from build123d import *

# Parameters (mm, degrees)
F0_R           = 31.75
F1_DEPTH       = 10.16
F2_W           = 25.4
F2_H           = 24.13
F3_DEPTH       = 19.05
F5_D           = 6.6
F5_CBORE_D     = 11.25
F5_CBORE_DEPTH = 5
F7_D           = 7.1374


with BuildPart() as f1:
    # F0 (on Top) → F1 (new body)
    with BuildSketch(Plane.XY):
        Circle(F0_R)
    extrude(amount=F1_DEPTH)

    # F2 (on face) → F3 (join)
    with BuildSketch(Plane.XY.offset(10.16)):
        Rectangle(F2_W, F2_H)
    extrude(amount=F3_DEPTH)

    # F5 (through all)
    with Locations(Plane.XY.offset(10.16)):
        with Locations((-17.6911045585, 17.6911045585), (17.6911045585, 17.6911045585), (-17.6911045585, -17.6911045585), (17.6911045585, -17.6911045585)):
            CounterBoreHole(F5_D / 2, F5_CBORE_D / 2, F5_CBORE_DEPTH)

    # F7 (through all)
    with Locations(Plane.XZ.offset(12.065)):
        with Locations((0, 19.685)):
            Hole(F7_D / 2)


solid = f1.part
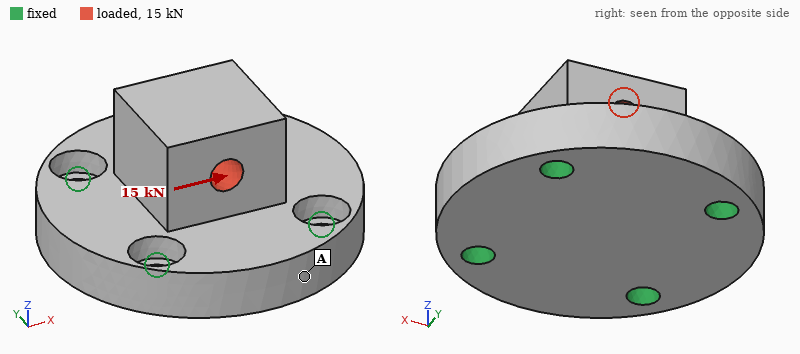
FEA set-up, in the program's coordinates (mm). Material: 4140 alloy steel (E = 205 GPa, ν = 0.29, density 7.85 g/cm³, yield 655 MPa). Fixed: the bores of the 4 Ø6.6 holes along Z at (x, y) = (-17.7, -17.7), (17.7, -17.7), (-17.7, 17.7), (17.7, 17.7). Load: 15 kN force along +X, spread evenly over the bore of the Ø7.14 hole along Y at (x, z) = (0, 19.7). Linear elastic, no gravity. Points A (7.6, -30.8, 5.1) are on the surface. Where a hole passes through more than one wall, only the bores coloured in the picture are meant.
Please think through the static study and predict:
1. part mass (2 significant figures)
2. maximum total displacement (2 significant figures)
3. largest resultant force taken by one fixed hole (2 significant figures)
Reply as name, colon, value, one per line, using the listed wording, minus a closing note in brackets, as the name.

part mass: 320 g
maximum total displacement: 21 µm
largest resultant force taken by one fixed hole: 5.6 kN
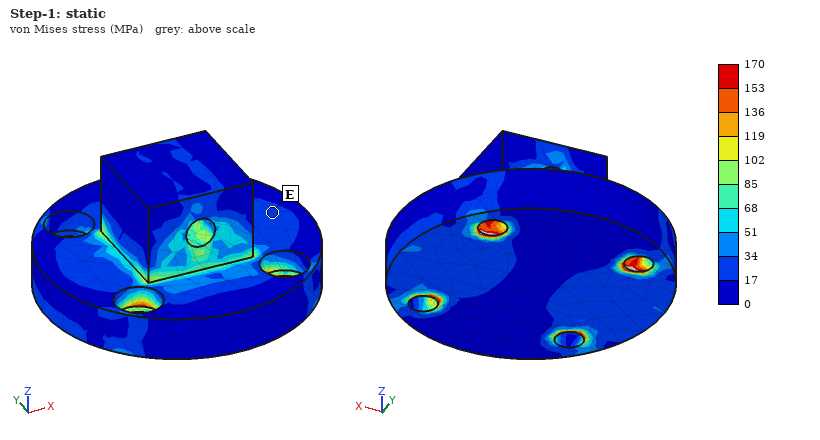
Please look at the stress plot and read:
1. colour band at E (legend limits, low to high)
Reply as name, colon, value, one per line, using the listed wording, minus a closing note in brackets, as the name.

colour band at E: 17 to 34 MPa
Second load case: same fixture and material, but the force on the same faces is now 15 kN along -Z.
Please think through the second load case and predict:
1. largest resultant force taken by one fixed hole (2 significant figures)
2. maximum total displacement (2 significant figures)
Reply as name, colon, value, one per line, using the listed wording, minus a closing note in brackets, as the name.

largest resultant force taken by one fixed hole: 4.4 kN
maximum total displacement: 9.9 µm
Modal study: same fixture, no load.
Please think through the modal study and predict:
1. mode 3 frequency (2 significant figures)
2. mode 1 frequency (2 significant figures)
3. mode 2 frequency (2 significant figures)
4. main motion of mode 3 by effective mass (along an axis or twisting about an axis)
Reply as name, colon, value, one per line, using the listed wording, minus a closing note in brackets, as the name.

mode 3 frequency: 17 kHz
mode 1 frequency: 15 kHz
mode 2 frequency: 15 kHz
main motion of mode 3 by effective mass: along Z
